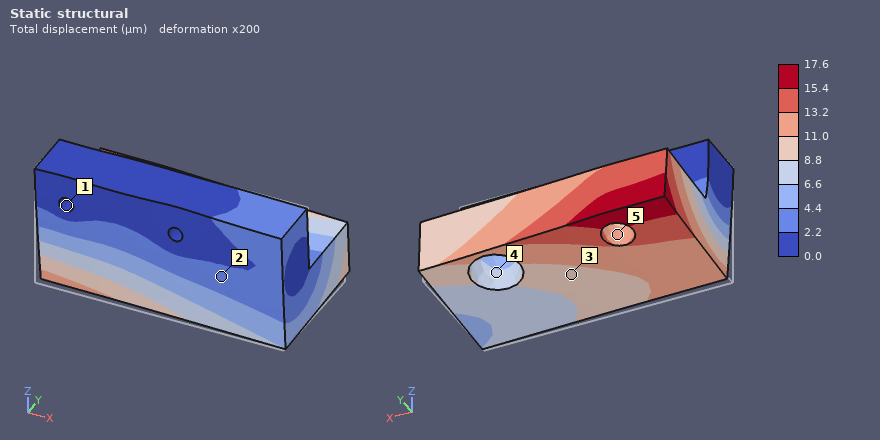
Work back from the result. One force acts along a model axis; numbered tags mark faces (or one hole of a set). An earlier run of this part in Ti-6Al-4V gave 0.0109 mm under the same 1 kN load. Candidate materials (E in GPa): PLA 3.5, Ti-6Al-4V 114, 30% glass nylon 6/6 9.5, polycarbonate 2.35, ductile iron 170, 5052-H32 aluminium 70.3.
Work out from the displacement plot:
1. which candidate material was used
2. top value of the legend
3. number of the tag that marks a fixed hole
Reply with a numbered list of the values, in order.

1. 5052-H32 aluminium
2. 17.6 µm
3. 1
